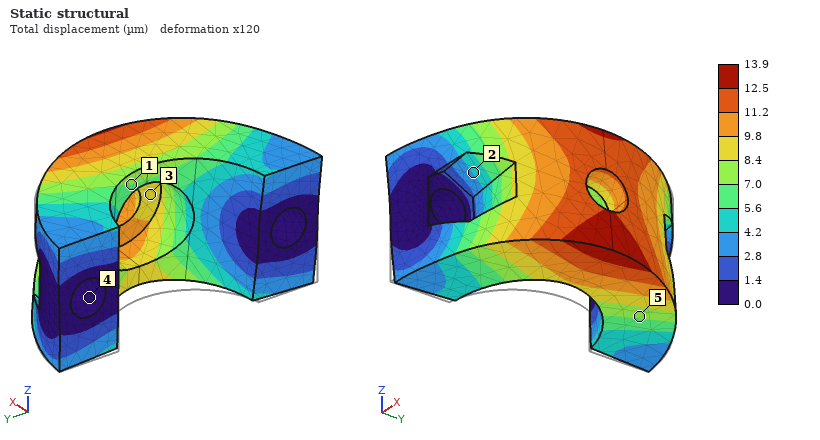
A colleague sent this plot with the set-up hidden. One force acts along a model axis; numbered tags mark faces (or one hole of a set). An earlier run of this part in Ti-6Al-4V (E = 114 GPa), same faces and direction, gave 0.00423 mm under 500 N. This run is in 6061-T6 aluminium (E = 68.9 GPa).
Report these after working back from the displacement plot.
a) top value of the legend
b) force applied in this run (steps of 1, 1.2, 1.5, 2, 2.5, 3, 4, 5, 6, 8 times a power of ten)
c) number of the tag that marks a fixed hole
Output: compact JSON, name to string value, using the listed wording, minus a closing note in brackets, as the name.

{"top value of the legend": "13.9 µm", "force applied in this run": "1 kN", "number of the tag that marks a fixed hole": "4"}
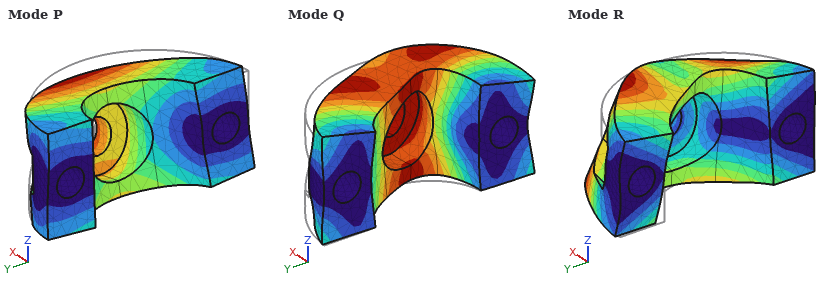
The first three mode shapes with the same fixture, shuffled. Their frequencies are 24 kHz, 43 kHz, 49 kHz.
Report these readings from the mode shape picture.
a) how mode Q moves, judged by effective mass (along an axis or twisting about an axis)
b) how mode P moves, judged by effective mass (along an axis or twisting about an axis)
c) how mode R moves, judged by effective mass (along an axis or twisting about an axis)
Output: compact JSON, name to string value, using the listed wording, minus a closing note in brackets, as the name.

{"how mode Q moves, judged by effective mass": "along Y", "how mode P moves, judged by effective mass": "along Z", "how mode R moves, judged by effective mass": "twisting about X"}
